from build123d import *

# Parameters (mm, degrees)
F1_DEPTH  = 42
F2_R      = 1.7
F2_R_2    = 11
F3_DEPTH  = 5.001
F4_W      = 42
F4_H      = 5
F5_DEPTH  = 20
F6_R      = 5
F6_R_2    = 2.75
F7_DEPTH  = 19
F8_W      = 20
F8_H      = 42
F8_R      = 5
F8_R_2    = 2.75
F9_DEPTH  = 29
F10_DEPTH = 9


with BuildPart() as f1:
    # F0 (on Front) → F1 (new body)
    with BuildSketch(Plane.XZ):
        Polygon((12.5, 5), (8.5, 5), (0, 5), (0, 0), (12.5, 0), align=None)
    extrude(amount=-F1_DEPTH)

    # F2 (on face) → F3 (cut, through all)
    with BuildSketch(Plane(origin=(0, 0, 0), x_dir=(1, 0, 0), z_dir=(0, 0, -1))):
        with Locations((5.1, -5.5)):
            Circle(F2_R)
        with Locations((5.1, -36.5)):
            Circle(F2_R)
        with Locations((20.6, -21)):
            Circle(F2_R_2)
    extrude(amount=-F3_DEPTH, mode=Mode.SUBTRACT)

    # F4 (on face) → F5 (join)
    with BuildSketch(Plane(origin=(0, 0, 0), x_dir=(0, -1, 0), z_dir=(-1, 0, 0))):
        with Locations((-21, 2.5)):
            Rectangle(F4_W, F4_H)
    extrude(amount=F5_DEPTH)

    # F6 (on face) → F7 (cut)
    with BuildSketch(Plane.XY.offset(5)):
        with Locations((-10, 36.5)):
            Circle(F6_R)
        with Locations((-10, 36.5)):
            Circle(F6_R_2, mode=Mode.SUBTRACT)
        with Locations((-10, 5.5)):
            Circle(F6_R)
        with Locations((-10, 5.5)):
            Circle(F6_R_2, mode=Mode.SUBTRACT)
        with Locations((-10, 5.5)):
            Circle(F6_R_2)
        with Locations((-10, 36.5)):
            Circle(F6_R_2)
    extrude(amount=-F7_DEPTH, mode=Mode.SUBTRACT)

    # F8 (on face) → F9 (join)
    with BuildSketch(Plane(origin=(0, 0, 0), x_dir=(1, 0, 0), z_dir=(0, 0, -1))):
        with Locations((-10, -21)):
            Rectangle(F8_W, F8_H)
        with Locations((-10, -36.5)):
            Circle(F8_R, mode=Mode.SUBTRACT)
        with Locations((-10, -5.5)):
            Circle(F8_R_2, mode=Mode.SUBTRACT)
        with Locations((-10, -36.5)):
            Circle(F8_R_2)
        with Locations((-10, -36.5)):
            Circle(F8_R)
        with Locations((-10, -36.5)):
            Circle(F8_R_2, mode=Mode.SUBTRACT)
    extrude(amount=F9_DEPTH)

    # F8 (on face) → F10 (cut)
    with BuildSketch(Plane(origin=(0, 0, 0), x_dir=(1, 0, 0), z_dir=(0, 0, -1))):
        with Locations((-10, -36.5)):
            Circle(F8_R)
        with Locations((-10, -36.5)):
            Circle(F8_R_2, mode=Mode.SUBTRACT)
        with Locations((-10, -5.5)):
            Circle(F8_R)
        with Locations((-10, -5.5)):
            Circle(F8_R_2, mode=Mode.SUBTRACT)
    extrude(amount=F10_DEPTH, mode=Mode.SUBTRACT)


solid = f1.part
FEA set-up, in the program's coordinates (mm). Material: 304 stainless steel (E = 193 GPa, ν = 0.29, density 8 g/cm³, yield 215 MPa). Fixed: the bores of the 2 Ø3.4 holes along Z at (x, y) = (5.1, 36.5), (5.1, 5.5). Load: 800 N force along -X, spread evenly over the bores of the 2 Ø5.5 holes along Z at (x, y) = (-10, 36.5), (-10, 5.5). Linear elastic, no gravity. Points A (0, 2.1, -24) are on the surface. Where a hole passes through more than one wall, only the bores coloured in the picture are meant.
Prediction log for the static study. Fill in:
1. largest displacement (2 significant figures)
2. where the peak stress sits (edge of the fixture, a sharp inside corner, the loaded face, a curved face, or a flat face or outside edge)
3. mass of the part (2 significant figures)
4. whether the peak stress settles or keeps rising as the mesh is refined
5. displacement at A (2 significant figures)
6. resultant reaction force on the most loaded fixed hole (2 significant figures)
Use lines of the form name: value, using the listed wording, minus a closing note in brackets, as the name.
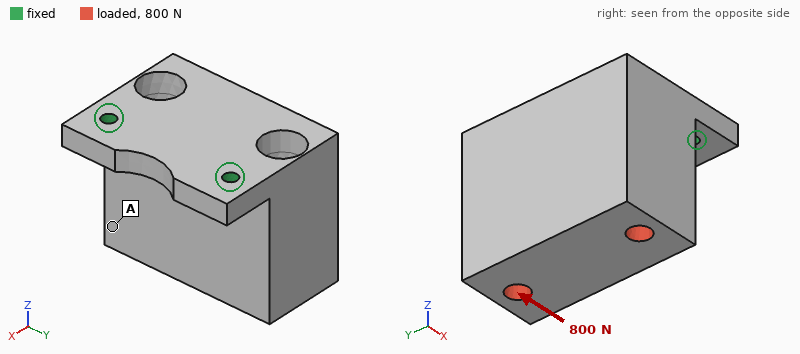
largest displacement: 78 µm
where the peak stress sits: edge of the fixture
mass of the part: 220 g
whether the peak stress settles or keeps rising as the mesh is refined: keeps rising
displacement at A: 54 µm
resultant reaction force on the most loaded fixed hole: 400 N
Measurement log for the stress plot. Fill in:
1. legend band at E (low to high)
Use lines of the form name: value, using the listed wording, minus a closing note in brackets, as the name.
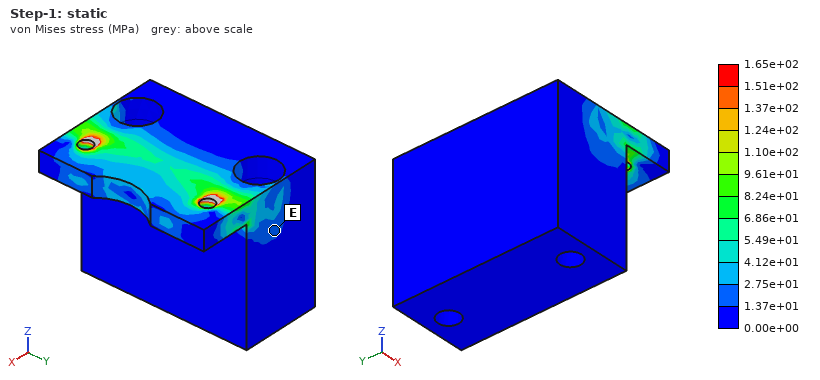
legend band at E: 1.37e+01 to 2.75e+01 MPa
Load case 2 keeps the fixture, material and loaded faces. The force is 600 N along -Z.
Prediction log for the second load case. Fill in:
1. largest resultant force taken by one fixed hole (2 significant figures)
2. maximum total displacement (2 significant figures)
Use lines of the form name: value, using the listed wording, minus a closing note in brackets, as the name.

largest resultant force taken by one fixed hole: 300 N
maximum total displacement: 32 µm
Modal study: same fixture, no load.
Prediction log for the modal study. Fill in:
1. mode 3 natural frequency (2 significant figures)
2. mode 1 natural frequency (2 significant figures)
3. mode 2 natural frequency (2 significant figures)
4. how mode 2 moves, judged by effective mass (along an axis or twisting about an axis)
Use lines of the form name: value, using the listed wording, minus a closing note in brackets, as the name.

mode 3 natural frequency: 9700 Hz
mode 1 natural frequency: 1500 Hz
mode 2 natural frequency: 5600 Hz
how mode 2 moves, judged by effective mass: along Y
